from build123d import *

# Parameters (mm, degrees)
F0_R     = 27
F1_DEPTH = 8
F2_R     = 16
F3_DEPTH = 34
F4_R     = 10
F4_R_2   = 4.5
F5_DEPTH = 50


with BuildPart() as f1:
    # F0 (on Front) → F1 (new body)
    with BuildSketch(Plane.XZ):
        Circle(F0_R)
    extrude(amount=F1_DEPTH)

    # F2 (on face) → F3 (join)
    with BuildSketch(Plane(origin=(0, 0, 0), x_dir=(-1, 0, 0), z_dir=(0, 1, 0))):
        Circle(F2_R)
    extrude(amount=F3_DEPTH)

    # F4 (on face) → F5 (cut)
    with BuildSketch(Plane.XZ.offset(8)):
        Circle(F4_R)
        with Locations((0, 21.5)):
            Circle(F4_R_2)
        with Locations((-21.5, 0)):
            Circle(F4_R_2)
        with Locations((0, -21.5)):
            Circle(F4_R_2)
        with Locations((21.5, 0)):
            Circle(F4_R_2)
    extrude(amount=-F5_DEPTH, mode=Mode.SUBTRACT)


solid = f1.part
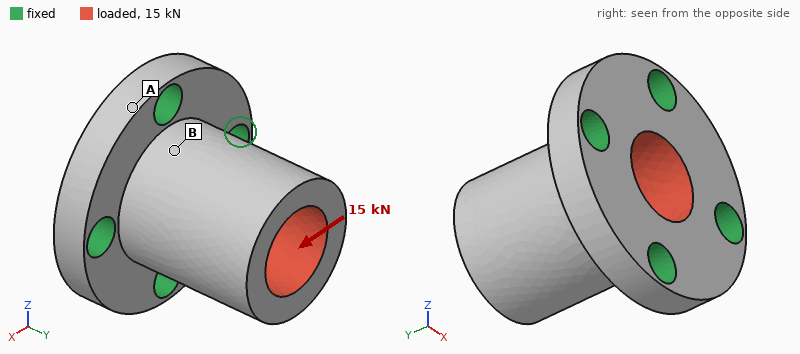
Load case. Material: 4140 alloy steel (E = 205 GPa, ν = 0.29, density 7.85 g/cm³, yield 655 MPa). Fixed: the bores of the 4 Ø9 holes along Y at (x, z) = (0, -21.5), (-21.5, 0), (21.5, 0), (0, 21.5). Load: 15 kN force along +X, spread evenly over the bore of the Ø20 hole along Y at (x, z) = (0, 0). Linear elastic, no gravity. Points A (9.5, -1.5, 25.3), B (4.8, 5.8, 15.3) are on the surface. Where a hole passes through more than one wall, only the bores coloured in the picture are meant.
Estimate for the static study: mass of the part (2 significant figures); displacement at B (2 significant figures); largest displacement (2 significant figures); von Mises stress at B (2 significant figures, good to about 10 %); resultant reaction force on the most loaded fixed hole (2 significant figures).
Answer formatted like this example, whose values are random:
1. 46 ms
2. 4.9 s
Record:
1. 240 g
2. 6.1 µm
3. 27 µm
4. 40 MPa
5. 8.0 kN
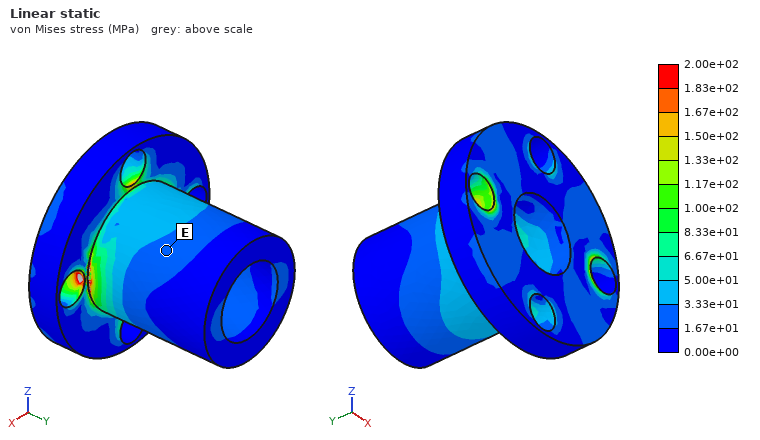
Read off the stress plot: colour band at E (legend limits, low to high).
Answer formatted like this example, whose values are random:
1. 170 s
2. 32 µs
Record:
1. 1.67e+01 to 3.33e+01 MPa
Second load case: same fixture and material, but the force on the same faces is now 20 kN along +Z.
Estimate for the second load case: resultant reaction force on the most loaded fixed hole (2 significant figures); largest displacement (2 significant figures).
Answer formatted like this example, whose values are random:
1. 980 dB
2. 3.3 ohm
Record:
1. 11 kN
2. 36 µm
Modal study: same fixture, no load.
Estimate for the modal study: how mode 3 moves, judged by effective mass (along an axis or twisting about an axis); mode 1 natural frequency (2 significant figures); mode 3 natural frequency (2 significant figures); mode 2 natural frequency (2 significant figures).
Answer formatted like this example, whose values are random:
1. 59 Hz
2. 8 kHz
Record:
1. twisting about Y
2. 11 kHz
3. 21 kHz
4. 11 kHz
